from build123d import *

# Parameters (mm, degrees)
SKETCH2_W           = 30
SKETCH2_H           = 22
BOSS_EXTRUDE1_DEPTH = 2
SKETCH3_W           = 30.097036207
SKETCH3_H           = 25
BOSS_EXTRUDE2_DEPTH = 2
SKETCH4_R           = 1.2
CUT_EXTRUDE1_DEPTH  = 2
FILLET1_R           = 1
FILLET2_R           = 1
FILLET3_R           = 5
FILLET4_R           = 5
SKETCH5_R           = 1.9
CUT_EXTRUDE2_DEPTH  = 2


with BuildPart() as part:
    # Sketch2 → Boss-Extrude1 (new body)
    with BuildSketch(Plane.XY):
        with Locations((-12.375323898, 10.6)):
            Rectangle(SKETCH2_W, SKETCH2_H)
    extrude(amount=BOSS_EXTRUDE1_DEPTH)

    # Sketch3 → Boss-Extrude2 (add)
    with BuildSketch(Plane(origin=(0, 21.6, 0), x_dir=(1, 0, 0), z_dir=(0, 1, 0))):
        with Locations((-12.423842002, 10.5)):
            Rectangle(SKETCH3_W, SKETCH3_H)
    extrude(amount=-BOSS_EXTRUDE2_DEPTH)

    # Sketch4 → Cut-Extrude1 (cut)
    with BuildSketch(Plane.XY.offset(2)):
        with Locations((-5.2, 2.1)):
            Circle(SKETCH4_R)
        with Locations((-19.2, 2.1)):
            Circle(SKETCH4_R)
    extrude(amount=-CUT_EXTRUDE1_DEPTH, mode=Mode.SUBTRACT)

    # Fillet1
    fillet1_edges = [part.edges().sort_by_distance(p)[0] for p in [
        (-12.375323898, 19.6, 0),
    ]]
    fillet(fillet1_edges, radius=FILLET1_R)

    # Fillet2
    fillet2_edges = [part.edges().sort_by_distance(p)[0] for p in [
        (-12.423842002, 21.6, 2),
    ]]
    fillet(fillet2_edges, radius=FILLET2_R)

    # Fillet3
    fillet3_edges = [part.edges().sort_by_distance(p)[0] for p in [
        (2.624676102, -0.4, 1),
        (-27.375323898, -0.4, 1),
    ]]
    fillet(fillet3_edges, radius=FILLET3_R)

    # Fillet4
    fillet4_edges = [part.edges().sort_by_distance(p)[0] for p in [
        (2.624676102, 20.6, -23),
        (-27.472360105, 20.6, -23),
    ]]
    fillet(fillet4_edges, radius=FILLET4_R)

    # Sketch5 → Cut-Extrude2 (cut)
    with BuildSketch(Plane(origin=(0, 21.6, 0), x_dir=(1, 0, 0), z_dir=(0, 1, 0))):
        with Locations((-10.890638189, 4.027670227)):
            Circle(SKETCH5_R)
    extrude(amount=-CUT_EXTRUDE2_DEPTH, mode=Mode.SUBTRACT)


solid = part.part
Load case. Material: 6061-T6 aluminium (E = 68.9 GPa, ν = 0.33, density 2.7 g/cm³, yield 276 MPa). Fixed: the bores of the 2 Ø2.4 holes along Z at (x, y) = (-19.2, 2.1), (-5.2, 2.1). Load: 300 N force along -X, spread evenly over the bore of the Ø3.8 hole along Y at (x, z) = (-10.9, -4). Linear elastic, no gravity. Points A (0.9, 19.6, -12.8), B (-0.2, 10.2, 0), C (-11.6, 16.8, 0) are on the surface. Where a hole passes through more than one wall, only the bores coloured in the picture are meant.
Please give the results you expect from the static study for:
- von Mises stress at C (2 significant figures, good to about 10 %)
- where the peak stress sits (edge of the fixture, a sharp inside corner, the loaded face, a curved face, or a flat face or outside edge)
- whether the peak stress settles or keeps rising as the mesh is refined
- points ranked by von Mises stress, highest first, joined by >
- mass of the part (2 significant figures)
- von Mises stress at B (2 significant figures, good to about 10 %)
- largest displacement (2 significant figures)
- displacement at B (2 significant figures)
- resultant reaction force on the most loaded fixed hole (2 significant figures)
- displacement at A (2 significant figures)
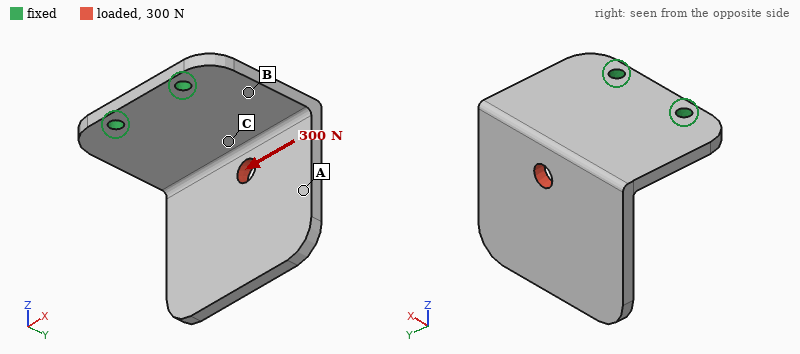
54 MPa
edge of the fixture
keeps rising
C > B > A
7.1 g
33 MPa
0.21 mm
0.037 mm
390 N
0.15 mm
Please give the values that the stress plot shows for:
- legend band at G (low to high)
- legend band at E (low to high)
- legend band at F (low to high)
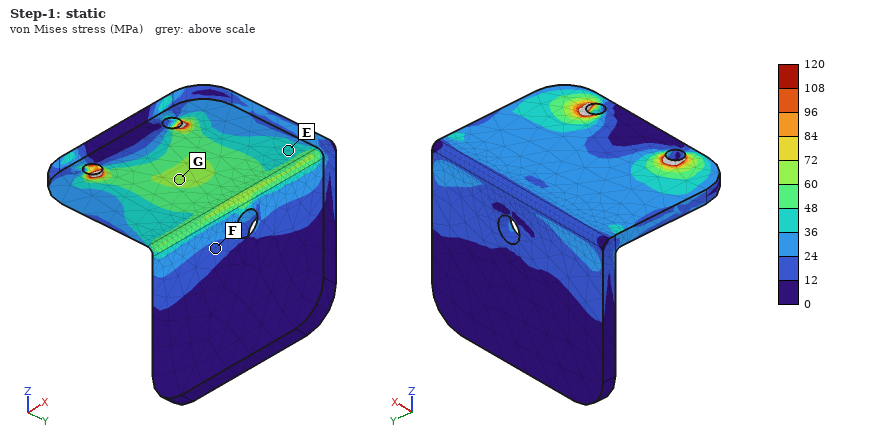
60 to 72 MPa
36 to 48 MPa
12 to 24 MPa
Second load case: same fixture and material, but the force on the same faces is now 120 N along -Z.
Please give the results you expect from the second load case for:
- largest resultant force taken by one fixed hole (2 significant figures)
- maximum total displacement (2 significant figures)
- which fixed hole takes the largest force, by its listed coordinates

69 N
0.42 mm
(-5.2, 2.1)
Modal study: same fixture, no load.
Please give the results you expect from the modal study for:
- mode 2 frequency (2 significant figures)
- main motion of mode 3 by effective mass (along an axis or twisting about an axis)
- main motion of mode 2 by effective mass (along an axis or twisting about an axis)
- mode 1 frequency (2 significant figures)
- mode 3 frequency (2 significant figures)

2200 Hz
along Z
along X
1200 Hz
3500 Hz
